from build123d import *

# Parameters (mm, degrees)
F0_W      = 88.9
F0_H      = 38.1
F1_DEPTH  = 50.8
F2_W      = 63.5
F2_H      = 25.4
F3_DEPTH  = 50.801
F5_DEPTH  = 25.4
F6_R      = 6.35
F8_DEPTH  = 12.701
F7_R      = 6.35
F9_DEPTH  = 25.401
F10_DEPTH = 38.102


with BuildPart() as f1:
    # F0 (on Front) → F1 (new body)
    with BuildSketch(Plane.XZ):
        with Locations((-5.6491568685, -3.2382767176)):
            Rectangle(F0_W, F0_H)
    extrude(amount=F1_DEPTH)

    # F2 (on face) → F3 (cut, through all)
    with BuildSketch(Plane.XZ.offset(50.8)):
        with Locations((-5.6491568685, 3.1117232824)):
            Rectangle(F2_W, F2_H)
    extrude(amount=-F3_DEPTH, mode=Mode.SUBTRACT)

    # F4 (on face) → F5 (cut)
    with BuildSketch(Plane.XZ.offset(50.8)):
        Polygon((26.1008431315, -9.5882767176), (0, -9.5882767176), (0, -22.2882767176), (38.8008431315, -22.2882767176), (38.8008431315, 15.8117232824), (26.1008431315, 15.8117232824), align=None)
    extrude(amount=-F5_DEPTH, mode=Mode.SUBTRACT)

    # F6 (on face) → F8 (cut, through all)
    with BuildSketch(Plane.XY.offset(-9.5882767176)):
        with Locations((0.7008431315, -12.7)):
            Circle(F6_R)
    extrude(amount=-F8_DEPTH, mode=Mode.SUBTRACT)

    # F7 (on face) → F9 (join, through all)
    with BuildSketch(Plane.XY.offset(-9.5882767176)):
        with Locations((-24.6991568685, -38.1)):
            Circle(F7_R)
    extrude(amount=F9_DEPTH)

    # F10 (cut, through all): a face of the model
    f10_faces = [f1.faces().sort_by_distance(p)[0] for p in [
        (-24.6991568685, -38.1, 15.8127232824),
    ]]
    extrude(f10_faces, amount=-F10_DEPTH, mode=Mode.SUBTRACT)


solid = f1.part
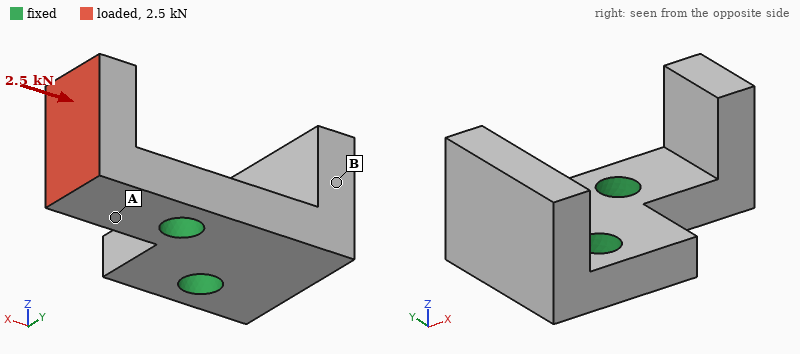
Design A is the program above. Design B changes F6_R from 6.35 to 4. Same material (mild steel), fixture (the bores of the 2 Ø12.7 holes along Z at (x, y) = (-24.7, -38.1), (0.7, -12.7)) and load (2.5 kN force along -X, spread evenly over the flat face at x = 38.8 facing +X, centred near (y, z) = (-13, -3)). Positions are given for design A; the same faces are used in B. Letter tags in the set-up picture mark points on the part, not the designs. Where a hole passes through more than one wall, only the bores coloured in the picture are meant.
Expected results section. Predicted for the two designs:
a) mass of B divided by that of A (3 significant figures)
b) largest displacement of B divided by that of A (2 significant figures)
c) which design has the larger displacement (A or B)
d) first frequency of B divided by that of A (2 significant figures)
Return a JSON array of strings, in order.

["1.01", "1.1", "B", "0.90"]
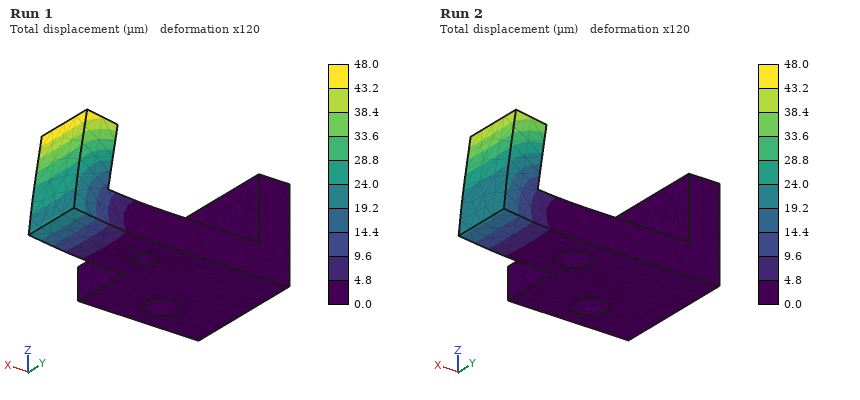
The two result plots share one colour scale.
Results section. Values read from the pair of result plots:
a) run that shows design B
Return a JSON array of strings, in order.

["Run 1"]
